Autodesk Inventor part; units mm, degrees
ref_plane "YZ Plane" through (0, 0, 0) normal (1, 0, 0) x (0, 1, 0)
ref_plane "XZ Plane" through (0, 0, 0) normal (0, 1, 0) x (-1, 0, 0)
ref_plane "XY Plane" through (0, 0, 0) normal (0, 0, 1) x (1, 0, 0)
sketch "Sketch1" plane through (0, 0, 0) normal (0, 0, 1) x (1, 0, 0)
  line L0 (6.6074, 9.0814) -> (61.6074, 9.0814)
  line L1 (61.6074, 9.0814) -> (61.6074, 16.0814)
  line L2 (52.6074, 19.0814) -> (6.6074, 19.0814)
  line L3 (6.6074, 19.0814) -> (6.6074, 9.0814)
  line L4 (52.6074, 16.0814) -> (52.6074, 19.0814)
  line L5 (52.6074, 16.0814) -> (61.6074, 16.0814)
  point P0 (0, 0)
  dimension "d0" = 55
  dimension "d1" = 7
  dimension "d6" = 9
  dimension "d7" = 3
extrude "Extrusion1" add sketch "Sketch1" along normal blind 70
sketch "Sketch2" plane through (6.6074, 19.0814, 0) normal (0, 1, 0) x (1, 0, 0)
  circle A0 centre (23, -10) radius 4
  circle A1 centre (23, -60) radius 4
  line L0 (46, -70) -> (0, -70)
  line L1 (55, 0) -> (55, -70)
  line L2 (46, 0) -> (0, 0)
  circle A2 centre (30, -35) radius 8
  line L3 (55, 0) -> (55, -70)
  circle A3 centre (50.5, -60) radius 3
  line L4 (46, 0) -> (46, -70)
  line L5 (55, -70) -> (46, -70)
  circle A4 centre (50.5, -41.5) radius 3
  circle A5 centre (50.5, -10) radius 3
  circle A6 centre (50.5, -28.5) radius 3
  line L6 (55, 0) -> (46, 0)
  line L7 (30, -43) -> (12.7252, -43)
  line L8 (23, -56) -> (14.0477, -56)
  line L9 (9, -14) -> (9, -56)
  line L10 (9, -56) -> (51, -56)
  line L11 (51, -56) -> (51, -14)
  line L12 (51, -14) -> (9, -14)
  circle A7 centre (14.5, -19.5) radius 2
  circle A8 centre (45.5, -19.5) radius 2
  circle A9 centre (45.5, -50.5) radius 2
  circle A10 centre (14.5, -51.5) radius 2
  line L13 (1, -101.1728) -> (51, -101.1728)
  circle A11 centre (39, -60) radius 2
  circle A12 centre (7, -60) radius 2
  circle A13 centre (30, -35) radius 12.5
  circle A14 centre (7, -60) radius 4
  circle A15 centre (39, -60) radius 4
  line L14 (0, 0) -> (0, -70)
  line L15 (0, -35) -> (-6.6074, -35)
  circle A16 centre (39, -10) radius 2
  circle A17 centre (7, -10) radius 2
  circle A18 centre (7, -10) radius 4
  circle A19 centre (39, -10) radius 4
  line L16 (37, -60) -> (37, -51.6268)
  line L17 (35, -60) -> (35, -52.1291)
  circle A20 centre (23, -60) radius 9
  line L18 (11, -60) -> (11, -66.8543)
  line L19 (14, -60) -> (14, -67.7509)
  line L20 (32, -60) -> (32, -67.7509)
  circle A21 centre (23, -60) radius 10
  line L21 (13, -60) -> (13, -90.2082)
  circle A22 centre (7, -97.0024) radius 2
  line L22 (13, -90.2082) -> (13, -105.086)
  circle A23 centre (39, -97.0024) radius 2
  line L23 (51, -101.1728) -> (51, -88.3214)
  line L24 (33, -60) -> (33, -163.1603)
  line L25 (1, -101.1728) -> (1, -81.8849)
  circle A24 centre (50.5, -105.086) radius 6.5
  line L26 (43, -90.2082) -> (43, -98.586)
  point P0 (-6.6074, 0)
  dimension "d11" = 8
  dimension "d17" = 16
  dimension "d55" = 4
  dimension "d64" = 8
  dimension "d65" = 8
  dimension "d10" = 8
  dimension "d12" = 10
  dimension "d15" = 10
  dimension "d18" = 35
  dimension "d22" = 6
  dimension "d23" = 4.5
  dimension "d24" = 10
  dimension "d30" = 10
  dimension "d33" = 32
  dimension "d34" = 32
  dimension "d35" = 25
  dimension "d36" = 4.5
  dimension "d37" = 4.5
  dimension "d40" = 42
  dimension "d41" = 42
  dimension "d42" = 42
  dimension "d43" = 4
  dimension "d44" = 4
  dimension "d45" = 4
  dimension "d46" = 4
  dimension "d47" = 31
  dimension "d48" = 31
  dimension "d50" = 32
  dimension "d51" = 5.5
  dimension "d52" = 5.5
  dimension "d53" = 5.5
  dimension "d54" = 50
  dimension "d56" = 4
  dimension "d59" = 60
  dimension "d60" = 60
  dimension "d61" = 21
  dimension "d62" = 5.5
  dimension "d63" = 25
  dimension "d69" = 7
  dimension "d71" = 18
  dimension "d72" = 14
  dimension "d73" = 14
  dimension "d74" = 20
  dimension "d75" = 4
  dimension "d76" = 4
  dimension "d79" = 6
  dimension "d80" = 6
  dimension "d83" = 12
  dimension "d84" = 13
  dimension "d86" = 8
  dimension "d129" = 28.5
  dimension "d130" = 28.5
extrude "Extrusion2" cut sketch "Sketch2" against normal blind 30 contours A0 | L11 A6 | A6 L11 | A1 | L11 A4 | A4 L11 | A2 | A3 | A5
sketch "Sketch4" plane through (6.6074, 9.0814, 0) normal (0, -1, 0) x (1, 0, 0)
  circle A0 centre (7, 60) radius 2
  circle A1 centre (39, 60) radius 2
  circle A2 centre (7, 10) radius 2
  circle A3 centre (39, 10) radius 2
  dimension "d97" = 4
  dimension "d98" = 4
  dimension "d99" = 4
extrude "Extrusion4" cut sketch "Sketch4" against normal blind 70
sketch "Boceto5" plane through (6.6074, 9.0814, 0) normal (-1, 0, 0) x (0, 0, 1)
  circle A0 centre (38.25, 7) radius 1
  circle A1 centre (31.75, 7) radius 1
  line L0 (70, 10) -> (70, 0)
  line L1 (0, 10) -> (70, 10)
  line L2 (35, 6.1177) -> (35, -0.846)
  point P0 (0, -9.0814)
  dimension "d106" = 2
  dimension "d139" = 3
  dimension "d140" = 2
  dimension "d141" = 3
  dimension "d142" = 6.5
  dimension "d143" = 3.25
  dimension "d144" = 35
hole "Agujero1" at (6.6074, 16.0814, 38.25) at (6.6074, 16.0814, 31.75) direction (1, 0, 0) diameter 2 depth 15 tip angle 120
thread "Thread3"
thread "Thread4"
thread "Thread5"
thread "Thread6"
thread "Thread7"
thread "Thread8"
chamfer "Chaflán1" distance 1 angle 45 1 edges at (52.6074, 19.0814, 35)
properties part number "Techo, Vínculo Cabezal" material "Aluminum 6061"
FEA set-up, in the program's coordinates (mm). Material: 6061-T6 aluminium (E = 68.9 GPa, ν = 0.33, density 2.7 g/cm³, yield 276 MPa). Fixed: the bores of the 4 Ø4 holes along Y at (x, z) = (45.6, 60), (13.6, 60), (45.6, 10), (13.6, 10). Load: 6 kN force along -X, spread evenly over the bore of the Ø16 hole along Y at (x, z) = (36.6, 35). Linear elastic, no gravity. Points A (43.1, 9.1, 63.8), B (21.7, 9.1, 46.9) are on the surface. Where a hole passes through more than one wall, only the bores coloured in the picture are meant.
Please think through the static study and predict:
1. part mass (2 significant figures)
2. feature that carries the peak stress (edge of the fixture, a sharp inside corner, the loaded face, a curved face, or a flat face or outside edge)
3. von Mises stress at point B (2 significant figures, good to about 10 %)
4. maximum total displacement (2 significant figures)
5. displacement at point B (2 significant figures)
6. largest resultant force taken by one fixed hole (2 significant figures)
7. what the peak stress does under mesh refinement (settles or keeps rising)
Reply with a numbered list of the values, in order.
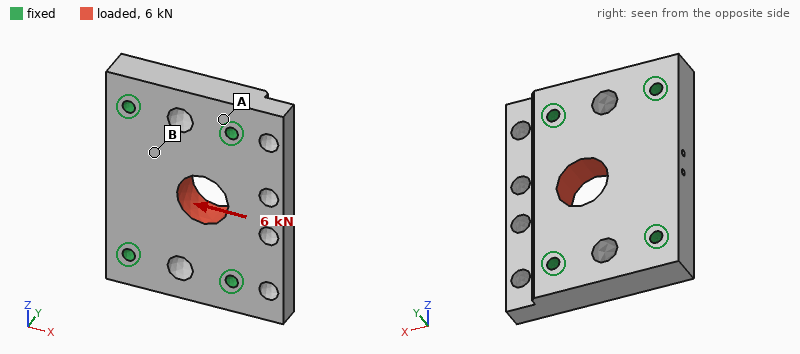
1. 87 g
2. edge of the fixture
3. 12 MPa
4. 10 µm
5. 4.1 µm
6. 1.7 kN
7. keeps rising
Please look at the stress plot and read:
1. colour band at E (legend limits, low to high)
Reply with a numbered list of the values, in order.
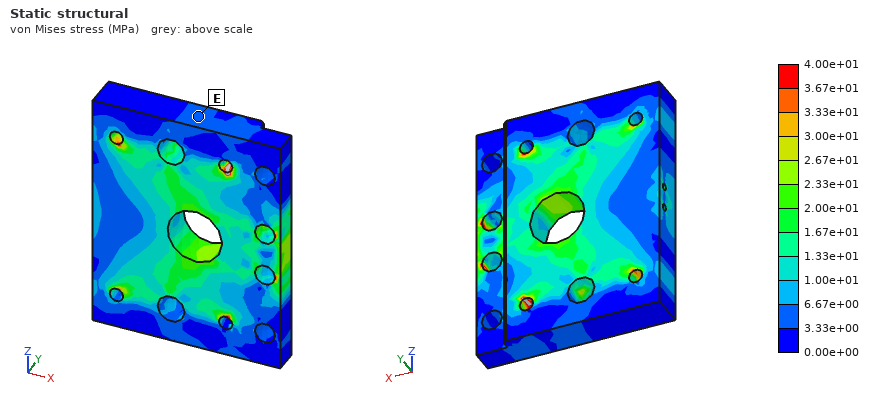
1. 3.33e+00 to 6.67e+00 MPa
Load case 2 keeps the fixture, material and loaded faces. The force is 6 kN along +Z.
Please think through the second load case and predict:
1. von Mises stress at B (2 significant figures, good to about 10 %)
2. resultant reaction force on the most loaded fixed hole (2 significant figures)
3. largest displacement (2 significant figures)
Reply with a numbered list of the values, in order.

1. 7.3 MPa
2. 2.0 kN
3. 4.1 µm
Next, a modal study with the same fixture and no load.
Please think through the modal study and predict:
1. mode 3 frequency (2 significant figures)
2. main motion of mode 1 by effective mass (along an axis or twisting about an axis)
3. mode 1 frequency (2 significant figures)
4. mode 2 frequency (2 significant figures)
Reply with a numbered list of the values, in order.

1. 24 kHz
2. along Y
3. 14 kHz
4. 16 kHz
